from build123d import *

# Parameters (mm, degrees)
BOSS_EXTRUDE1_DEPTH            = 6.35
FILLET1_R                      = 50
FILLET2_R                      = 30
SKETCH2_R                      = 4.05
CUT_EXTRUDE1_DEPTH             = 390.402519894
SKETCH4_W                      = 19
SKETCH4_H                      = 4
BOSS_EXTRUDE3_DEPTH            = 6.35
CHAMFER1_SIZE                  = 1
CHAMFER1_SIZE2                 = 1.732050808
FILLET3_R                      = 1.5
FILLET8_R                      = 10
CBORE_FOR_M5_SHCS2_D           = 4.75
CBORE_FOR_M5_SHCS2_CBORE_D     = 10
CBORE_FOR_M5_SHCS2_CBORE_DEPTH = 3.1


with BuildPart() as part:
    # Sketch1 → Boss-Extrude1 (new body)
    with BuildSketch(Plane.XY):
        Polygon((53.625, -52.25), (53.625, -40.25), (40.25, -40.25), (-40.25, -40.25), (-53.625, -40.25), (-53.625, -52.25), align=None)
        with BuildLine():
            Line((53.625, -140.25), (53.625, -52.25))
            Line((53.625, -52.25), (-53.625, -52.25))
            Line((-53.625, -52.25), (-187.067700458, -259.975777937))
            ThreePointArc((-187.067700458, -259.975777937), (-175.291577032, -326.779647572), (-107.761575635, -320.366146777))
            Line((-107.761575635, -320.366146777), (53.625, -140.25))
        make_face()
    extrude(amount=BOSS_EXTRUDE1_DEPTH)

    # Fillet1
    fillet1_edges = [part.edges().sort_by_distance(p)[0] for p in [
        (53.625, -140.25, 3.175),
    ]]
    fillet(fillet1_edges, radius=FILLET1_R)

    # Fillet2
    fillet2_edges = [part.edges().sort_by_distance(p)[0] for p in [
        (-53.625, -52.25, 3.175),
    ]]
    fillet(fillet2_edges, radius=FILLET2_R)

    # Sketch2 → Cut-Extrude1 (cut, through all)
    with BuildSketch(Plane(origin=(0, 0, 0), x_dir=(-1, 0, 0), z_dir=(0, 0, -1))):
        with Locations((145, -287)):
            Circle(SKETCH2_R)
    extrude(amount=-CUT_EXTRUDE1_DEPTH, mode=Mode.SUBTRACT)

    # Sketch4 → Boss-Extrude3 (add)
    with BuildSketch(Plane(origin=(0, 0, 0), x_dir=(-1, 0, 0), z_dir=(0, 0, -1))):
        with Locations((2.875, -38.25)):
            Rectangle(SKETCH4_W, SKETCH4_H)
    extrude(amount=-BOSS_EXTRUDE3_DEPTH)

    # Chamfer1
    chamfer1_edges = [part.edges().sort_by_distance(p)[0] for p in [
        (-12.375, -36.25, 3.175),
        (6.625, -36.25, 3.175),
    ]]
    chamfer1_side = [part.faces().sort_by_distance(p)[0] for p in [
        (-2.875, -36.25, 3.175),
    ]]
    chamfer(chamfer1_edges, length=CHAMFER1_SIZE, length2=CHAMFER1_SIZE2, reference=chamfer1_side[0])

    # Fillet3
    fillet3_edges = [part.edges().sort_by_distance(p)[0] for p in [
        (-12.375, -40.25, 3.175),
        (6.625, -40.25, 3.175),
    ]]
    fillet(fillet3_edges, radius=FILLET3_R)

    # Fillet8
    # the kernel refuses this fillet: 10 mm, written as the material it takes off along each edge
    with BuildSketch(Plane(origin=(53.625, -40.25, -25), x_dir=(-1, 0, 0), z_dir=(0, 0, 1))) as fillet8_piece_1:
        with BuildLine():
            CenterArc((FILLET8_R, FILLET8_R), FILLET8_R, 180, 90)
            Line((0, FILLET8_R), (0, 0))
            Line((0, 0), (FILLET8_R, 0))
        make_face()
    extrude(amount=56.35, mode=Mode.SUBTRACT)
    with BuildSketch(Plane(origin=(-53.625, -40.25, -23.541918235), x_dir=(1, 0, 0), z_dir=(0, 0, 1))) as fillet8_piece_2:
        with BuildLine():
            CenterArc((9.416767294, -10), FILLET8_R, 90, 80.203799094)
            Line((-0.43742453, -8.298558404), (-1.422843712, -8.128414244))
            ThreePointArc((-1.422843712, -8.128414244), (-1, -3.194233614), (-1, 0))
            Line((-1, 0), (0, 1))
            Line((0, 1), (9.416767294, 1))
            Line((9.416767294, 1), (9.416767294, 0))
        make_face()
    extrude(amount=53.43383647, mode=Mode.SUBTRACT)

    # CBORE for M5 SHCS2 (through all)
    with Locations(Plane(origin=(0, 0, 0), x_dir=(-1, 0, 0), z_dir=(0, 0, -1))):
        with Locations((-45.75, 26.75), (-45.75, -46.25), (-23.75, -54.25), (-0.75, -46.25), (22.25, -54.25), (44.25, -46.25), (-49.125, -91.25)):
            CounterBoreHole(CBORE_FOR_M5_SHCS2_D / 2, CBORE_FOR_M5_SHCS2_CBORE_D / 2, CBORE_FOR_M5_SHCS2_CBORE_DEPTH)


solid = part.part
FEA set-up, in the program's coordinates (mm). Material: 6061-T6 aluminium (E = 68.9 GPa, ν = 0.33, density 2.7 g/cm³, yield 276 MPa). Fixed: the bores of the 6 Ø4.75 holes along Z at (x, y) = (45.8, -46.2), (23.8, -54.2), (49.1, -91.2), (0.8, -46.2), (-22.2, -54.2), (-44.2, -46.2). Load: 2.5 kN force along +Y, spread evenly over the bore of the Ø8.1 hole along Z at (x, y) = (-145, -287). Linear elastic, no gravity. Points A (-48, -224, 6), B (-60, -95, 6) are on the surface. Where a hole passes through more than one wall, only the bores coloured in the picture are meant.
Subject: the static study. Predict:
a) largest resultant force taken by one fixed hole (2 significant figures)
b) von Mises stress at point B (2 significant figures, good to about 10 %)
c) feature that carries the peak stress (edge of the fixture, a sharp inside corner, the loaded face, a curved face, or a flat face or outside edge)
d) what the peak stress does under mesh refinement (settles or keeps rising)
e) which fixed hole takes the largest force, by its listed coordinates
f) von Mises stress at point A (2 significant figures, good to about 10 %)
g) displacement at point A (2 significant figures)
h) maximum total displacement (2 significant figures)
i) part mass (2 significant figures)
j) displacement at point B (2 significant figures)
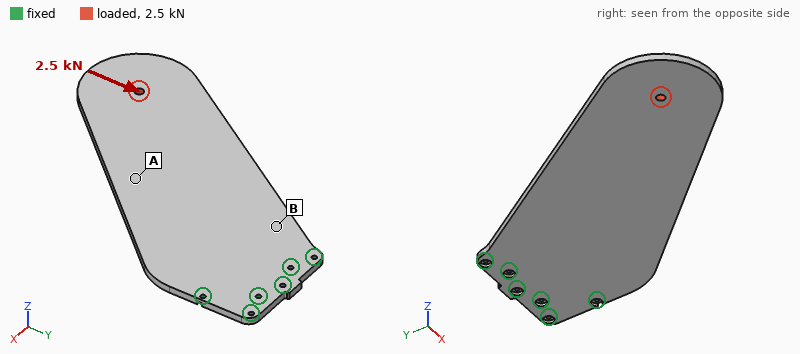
3.0 kN
18 MPa
edge of the fixture
keeps rising
(-44.2, -46.2)
5.5 MPa
0.090 mm
0.25 mm
660 g
0.048 mm
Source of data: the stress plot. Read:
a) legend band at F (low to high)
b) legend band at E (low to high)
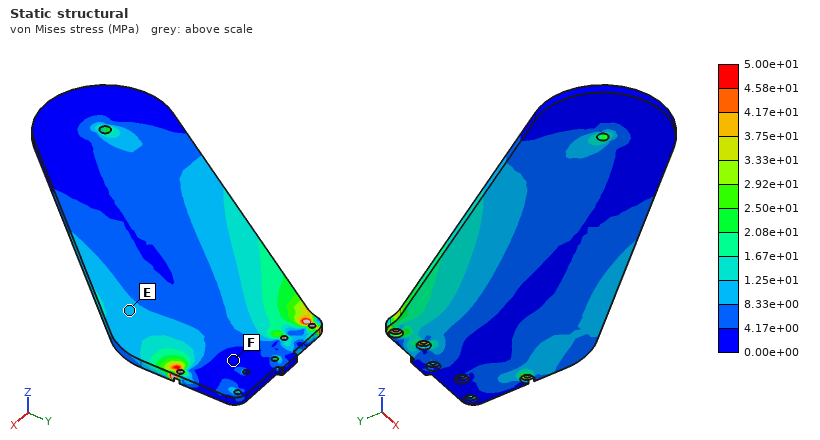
0.00e+00 to 4.17e+00 MPa
8.33e+00 to 1.25e+01 MPa
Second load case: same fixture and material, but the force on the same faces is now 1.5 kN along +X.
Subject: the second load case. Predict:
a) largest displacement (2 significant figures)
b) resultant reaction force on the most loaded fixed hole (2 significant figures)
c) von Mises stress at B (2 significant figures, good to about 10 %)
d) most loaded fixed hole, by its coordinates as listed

0.19 mm
2.9 kN
12 MPa
(49.1, -91.2)
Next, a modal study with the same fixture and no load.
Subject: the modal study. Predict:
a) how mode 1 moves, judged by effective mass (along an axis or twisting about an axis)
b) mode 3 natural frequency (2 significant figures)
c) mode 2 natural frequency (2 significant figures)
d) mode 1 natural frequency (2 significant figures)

along Z
360 Hz
310 Hz
58 Hz
